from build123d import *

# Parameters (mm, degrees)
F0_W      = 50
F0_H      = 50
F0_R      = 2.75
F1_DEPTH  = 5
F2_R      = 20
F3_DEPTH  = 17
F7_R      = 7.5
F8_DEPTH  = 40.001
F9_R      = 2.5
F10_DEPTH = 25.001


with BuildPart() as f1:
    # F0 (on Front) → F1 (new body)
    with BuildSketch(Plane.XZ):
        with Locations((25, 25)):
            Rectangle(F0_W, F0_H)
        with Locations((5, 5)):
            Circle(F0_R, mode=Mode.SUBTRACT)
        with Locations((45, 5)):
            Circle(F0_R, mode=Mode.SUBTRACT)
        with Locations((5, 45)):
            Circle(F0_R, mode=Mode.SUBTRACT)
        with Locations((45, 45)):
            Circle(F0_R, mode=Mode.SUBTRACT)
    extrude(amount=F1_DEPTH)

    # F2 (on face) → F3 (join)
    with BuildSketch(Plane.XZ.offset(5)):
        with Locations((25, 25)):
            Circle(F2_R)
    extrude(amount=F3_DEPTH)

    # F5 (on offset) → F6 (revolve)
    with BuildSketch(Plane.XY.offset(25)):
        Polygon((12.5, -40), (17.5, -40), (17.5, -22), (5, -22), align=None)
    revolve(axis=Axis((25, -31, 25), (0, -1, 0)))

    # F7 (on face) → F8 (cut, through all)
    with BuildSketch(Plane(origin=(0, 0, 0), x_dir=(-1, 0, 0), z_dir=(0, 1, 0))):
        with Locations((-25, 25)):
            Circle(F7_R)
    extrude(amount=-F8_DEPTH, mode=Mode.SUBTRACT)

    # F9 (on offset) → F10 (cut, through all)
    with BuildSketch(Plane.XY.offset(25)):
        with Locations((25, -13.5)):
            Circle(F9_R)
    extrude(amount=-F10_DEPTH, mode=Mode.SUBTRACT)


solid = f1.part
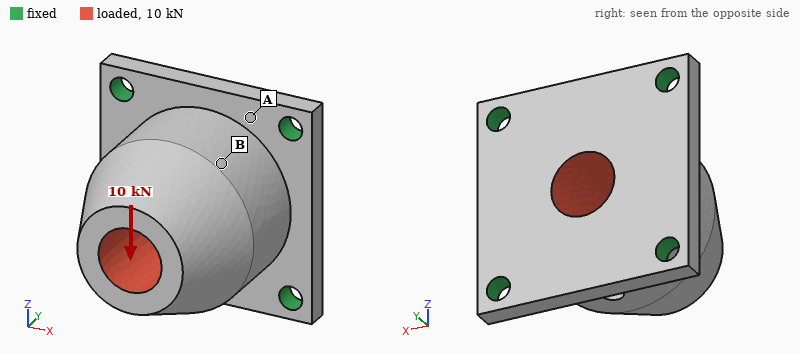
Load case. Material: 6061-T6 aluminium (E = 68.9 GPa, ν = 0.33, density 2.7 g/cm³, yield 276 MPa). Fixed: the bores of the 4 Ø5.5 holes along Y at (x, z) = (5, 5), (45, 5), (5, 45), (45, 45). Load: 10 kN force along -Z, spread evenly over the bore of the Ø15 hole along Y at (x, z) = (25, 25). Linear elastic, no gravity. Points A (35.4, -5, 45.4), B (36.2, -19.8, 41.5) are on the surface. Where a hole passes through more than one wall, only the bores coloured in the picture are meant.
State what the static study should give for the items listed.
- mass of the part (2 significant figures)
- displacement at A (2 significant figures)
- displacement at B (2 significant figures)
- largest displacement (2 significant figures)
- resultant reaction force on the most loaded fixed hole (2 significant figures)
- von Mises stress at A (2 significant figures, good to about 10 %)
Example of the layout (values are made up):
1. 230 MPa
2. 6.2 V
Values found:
1. 110 g
2. 24 µm
3. 51 µm
4. 86 µm
5. 3.8 kN
6. 60 MPa
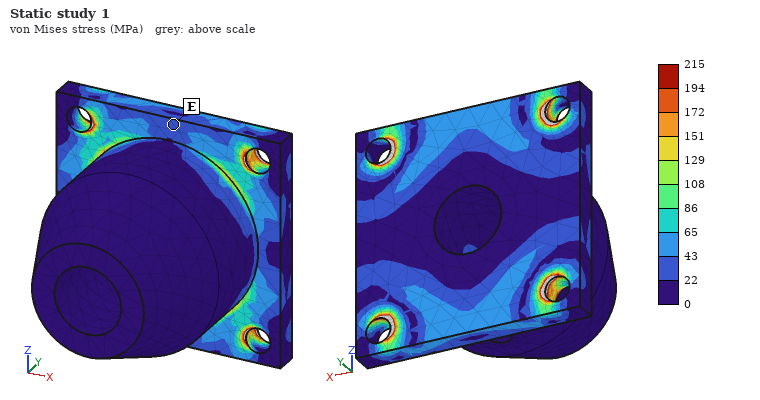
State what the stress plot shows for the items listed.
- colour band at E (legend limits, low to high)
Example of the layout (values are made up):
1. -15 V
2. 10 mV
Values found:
1. 22 to 43 MPa
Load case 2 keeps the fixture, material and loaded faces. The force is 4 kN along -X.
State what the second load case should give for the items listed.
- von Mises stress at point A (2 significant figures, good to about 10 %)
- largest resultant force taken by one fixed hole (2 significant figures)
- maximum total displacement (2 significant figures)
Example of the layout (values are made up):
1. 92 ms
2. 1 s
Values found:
1. 26 MPa
2. 1.5 kN
3. 35 µm
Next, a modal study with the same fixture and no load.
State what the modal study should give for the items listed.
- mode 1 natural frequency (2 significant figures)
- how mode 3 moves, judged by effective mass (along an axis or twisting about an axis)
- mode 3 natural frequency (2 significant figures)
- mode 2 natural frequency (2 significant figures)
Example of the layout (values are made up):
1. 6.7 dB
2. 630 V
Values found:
1. 7100 Hz
2. along Y
3. 9000 Hz
4. 7100 Hz
